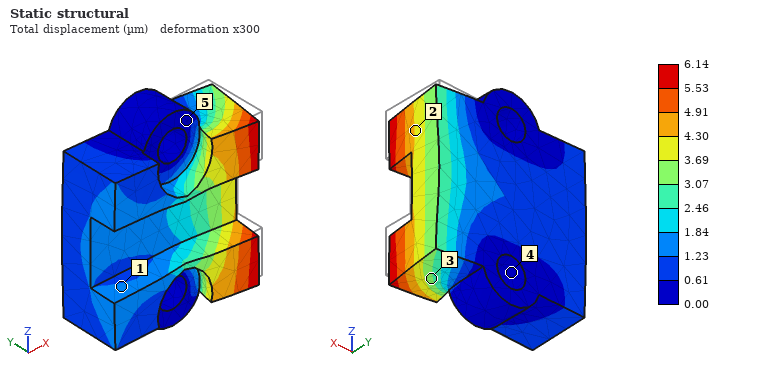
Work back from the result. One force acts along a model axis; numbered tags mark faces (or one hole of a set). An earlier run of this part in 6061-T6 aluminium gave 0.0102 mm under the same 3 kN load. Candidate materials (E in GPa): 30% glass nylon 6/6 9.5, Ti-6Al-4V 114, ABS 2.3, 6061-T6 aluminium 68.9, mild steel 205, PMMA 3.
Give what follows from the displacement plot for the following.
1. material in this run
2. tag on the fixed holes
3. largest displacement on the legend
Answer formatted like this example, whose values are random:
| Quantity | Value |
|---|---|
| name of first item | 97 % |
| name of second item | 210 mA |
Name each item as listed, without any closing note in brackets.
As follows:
| Quantity | Value |
|---|---|
| material in this run | Ti-6Al-4V |
| tag on the fixed holes | 4 |
| largest displacement on the legend | 6.14 µm |
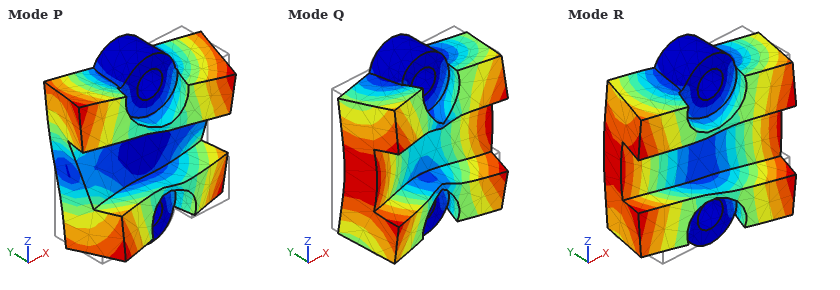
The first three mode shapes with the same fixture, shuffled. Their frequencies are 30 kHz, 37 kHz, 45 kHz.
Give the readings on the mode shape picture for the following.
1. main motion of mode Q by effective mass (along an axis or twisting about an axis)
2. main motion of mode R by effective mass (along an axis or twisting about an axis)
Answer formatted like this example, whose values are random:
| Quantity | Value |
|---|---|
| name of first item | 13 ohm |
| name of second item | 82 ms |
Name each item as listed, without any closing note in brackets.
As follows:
| Quantity | Value |
|---|---|
| main motion of mode Q by effective mass | along Y |
| main motion of mode R by effective mass | twisting about Z |
